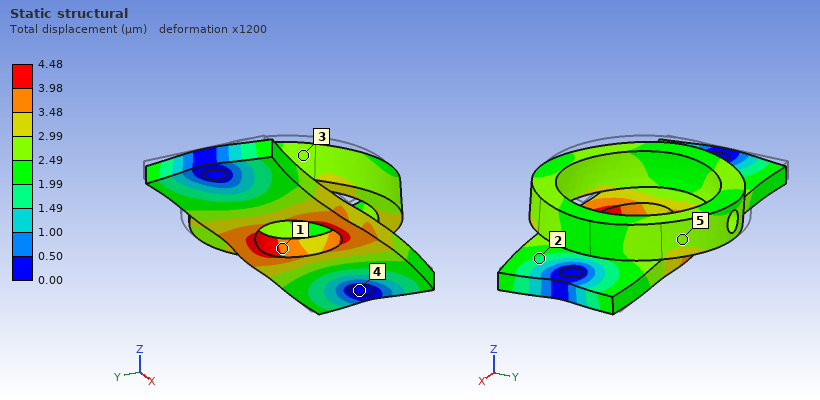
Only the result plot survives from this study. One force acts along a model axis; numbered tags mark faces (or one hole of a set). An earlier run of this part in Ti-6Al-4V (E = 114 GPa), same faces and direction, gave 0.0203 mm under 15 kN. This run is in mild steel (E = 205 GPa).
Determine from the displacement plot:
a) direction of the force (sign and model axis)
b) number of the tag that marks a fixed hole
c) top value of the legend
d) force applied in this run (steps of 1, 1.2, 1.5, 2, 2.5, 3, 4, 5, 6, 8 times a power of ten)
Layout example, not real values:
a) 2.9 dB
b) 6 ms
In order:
a) +X
b) 4
c) 4.48 µm
d) 6 kN
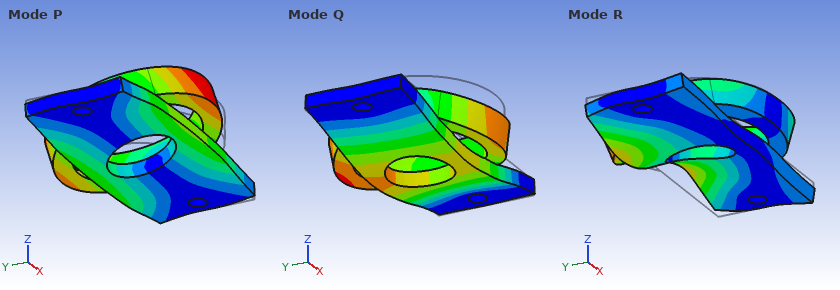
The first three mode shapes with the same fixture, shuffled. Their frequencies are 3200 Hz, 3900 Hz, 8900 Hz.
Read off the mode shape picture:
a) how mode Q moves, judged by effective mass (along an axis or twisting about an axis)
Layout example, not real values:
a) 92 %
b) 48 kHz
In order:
a) along Z
